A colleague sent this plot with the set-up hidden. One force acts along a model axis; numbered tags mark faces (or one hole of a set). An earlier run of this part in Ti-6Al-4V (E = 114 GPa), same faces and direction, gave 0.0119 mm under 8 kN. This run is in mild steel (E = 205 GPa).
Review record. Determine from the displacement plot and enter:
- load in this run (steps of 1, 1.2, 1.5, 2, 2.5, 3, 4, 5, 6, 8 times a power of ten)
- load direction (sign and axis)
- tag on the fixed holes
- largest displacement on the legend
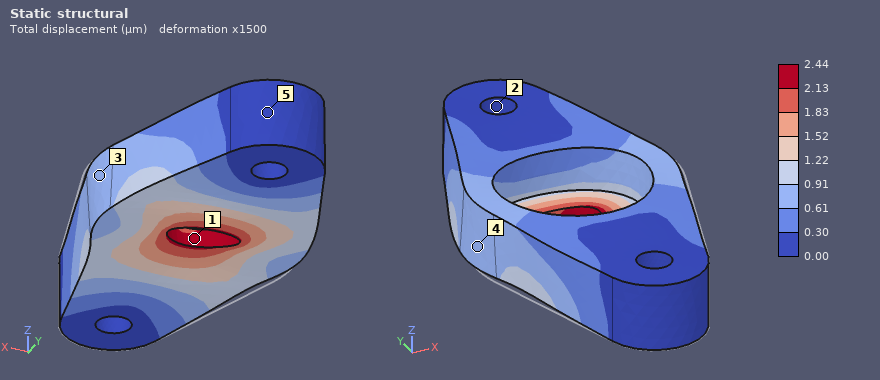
3 kN
+Y
2
2.44 µm
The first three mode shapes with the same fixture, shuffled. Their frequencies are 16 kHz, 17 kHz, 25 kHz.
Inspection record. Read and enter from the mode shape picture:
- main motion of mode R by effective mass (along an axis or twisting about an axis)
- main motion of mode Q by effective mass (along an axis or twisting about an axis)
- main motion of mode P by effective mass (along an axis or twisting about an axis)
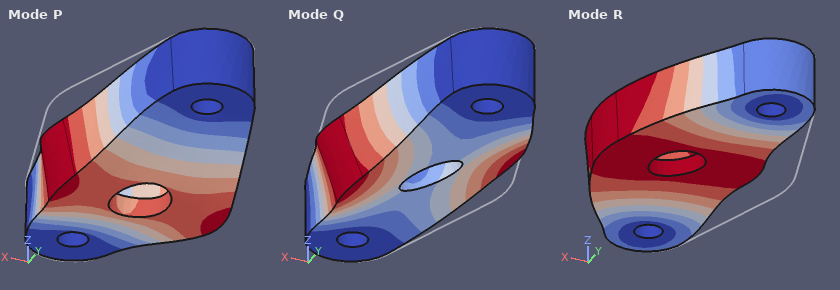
along X
twisting about Y
along Z
